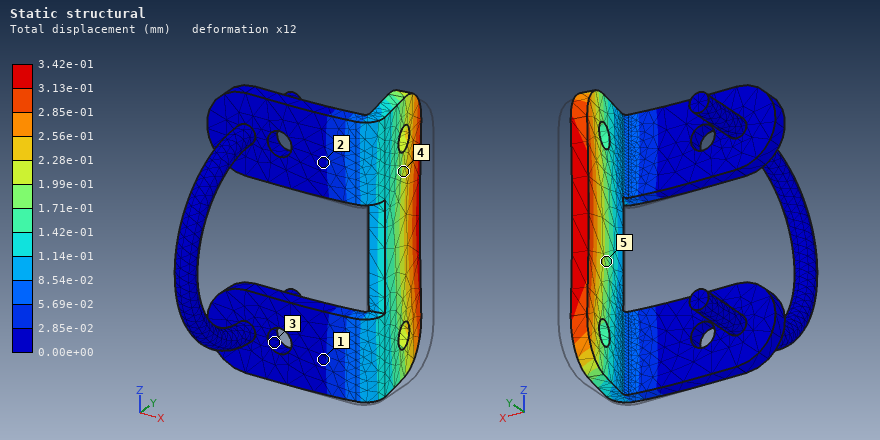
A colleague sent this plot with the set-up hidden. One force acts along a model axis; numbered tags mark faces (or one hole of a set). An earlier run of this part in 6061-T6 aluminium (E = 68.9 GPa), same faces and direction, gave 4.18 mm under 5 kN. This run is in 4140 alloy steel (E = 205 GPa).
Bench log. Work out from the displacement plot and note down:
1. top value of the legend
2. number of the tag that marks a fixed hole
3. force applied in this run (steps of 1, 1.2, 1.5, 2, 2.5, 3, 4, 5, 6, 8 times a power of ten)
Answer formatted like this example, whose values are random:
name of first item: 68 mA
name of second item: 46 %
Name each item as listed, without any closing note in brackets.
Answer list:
top value of the legend: 3.42e-01 mm
number of the tag that marks a fixed hole: 3
force applied in this run: 1.2 kN
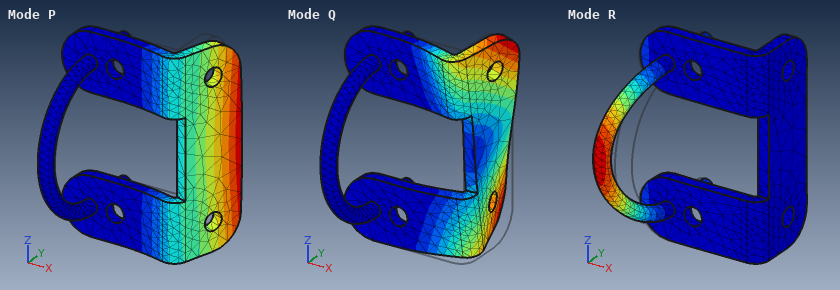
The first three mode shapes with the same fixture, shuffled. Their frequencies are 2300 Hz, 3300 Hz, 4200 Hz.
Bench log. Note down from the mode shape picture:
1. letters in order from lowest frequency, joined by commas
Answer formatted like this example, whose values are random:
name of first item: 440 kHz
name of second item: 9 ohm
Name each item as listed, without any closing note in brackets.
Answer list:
letters in order from lowest frequency, joined by commas: P, R, Q
